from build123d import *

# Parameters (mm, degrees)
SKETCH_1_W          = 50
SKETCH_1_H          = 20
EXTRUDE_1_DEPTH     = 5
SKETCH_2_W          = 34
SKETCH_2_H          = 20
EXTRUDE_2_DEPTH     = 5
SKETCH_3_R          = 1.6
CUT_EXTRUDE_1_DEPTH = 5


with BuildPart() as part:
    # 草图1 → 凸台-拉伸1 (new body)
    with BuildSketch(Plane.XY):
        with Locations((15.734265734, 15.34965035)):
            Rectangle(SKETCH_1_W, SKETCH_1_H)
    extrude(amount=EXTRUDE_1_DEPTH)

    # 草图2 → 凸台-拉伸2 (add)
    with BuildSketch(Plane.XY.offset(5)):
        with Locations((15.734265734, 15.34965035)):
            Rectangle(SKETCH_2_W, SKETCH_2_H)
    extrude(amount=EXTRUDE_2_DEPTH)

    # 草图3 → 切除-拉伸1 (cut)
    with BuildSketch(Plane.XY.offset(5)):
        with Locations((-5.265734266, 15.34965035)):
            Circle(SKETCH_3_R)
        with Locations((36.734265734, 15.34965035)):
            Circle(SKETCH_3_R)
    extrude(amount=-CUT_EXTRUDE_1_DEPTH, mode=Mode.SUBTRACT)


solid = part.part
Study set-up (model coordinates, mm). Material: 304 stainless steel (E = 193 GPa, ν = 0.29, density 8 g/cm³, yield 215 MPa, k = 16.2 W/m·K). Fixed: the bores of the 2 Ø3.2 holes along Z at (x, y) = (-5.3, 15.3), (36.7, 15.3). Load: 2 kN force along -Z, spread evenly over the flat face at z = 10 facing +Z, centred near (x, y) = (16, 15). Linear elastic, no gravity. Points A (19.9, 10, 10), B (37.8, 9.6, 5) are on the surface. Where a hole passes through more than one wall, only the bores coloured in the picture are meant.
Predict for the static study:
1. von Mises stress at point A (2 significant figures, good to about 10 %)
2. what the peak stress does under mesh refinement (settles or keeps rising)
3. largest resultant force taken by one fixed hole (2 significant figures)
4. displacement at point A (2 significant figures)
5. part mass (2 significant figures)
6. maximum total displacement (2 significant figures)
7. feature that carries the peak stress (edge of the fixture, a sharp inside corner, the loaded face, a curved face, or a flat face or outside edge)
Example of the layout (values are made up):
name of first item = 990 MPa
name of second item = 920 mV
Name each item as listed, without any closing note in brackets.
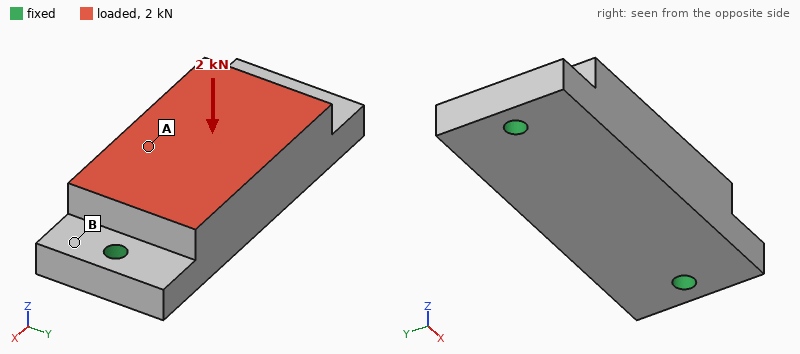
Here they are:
von Mises stress at point A = 22 MPa
what the peak stress does under mesh refinement = keeps rising
largest resultant force taken by one fixed hole = 1.2 kN
displacement at point A = 5.2 µm
part mass = 67 g
maximum total displacement = 5.6 µm
feature that carries the peak stress = edge of the fixture
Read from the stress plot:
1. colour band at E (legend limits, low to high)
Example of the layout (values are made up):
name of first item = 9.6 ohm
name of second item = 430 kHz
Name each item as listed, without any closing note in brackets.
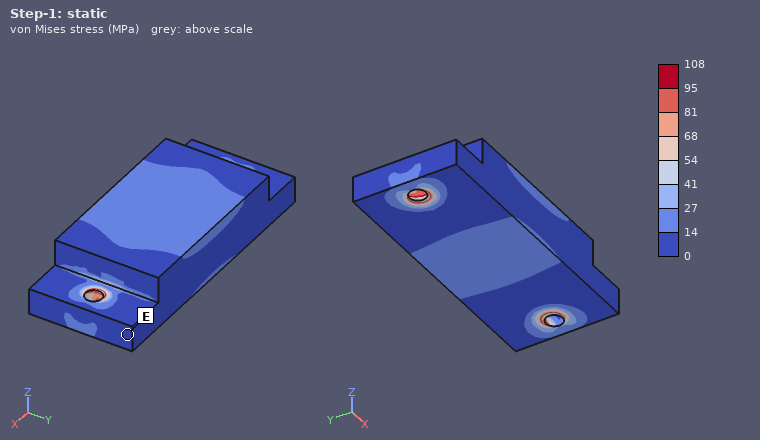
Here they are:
colour band at E = 0 to 14 MPa
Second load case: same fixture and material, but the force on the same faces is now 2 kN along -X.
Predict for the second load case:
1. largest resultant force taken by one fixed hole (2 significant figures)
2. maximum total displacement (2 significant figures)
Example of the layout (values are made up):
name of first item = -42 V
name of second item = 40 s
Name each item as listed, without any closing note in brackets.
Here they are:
largest resultant force taken by one fixed hole = 1.1 kN
maximum total displacement = 1.5 µm
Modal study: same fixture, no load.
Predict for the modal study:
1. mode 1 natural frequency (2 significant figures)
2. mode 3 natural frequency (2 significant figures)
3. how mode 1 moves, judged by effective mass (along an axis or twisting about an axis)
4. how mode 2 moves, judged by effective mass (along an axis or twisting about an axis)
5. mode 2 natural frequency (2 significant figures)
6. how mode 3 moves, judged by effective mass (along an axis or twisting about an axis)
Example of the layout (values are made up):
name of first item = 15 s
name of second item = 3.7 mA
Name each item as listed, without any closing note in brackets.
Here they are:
mode 1 natural frequency = 11 kHz
mode 3 natural frequency = 20 kHz
how mode 1 moves, judged by effective mass = along Y
how mode 2 moves, judged by effective mass = along Z
mode 2 natural frequency = 14 kHz
how mode 3 moves, judged by effective mass = along Y
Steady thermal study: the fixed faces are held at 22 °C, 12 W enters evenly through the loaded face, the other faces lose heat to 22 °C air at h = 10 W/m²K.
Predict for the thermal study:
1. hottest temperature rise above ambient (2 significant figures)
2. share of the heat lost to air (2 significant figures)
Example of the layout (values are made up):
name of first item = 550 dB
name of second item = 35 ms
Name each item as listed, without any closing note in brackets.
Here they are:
hottest temperature rise above ambient = 46 K
share of the heat lost to air = 5.6 %
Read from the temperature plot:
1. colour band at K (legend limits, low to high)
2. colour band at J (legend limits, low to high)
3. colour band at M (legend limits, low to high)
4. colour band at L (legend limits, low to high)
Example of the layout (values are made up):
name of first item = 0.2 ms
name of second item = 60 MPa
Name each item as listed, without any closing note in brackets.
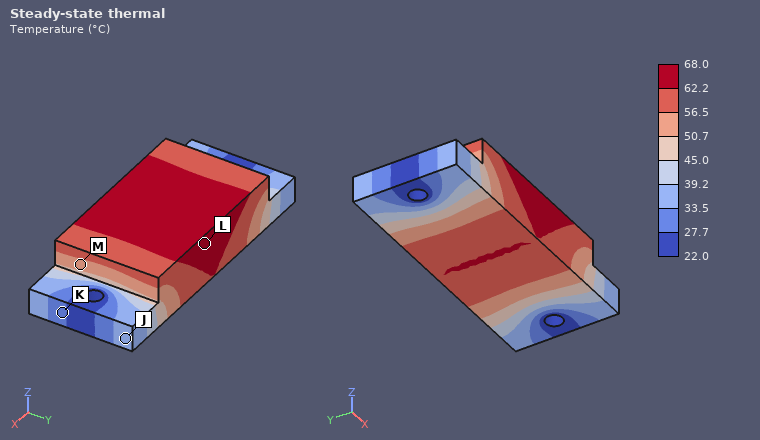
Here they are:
colour band at K = 27.7 to 33.5 °C
colour band at J = 33.5 to 39.2 °C
colour band at M = 50.7 to 56.5 °C
colour band at L = 62.2 to 68.0 °C
